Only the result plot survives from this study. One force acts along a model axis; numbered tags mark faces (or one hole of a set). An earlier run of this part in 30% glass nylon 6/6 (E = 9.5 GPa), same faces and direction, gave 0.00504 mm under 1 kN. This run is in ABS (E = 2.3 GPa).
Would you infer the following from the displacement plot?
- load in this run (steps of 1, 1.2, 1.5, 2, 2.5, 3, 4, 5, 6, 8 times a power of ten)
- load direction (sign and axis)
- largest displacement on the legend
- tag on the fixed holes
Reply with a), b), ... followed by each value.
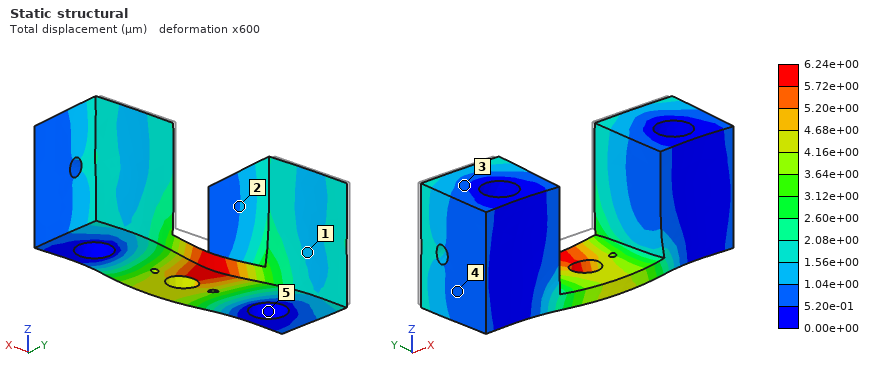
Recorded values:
a) 300 N
b) -Y
c) 6.24e+00 µm
d) 5
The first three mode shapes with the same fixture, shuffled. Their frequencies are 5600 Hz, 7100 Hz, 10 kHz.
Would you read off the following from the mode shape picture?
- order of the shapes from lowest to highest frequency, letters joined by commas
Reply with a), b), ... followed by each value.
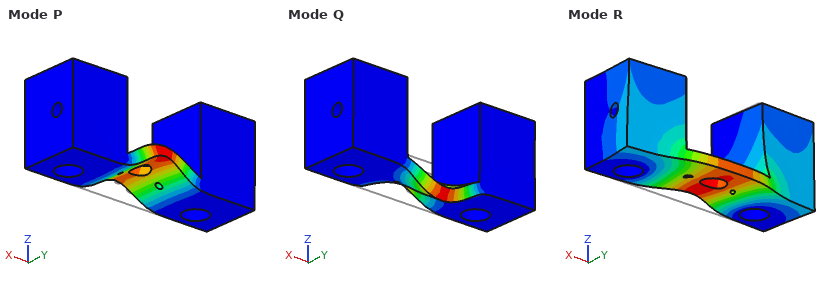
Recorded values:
a) P, Q, R
